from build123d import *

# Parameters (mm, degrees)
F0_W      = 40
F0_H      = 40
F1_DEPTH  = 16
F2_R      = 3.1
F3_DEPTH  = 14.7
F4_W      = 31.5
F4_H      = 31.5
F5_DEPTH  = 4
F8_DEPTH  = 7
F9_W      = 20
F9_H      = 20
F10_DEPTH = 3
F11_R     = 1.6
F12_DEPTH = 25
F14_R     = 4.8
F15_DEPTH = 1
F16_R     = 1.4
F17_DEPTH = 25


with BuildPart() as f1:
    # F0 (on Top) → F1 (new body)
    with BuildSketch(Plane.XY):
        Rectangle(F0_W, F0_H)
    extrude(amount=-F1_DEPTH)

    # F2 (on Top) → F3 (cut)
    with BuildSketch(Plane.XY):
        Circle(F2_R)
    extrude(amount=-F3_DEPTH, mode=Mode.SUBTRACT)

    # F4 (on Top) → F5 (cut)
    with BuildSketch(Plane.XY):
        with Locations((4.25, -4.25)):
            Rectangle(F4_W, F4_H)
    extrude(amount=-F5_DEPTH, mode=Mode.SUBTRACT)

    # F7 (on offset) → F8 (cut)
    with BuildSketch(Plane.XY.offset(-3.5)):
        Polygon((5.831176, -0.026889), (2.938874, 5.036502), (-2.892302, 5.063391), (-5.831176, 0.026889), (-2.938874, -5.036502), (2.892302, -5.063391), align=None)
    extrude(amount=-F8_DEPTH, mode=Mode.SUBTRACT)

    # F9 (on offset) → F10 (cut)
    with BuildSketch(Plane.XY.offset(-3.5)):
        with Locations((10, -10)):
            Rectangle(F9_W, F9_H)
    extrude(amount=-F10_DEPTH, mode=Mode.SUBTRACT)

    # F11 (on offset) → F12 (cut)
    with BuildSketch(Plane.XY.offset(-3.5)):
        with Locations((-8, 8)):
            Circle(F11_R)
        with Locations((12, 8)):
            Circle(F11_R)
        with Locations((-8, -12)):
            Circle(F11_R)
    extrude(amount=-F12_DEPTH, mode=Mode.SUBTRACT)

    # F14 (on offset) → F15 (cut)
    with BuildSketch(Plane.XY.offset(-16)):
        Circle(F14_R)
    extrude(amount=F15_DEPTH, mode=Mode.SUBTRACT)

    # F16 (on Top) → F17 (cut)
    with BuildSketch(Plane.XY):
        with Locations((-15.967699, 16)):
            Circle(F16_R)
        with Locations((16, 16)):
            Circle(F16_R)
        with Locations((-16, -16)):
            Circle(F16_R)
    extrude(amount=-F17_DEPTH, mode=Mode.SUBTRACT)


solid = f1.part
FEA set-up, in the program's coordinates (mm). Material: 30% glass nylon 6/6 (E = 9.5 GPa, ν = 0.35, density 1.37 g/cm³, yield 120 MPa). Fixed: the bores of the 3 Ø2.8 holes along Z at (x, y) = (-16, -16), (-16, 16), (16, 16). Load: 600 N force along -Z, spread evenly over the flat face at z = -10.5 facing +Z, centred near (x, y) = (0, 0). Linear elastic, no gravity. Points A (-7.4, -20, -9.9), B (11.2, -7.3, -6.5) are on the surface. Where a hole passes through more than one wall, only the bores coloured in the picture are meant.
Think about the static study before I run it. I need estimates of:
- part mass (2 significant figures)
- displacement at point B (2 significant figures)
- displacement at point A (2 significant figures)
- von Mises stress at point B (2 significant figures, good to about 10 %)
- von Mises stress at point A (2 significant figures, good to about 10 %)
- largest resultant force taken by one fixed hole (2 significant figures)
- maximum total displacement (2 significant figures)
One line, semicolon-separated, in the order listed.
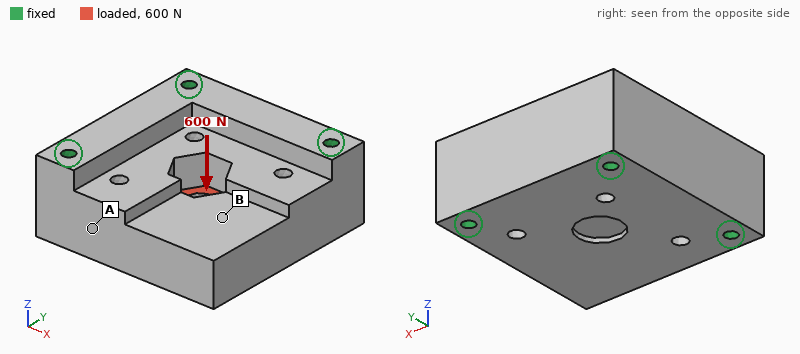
26 g; 18 µm; 4.5 µm; 3.5 MPa; 2.0 MPa; 240 N; 25 µm
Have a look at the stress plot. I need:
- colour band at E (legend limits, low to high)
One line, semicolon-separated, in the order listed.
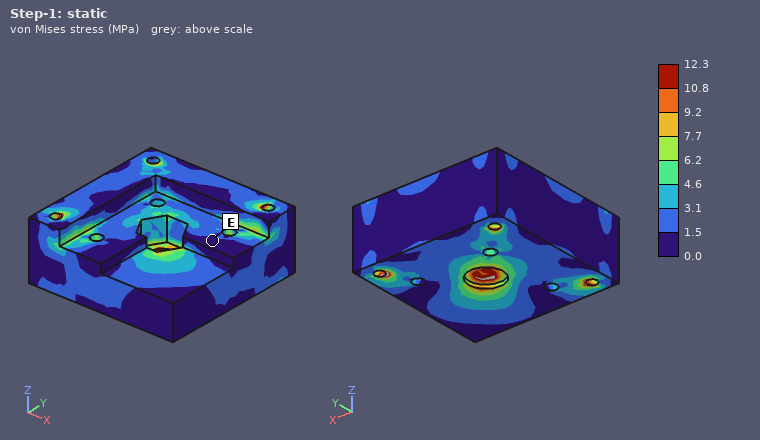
0.0 to 1.5 MPa
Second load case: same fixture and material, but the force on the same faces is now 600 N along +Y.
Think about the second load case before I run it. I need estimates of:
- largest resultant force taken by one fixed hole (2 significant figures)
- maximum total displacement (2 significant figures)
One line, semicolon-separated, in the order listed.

240 N; 11 µm
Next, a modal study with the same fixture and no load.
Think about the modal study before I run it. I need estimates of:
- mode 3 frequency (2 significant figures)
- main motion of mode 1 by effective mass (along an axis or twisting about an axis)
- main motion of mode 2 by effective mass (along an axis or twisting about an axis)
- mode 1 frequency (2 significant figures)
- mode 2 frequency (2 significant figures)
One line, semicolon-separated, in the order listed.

16 kHz; along Z; along Z; 6200 Hz; 15 kHz
